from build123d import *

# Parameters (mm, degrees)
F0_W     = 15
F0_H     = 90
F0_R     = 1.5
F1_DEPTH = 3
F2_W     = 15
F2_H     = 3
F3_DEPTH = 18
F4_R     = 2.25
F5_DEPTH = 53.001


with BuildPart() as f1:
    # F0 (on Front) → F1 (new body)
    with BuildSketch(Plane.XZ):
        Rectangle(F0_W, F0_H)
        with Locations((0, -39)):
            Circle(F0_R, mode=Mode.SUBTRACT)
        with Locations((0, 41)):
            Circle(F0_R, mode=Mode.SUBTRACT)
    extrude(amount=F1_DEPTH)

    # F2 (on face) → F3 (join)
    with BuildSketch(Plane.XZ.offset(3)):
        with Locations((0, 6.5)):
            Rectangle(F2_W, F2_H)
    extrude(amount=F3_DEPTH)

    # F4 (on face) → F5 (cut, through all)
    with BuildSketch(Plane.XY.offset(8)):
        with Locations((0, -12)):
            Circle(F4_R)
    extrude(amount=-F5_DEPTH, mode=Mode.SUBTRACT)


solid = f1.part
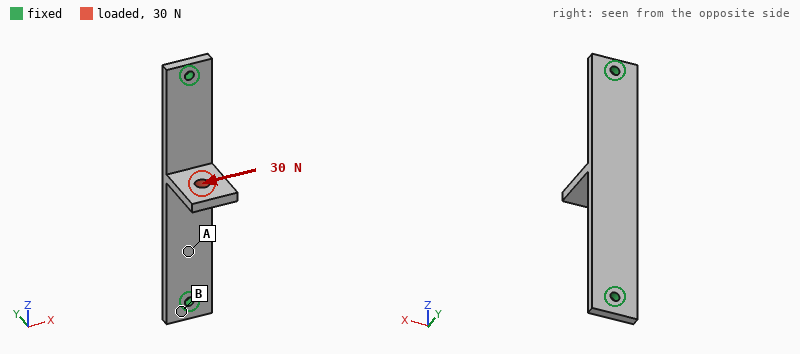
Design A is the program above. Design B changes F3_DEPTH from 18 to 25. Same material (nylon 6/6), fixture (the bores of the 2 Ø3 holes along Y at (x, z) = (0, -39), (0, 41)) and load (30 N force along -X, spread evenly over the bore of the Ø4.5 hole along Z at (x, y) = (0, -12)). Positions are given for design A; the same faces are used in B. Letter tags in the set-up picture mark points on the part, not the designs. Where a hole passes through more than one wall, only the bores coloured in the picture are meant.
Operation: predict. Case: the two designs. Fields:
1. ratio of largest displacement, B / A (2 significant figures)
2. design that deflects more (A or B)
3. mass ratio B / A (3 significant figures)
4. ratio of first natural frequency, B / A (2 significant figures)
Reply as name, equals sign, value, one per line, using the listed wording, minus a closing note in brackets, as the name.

ratio of largest displacement, B / A = 1.3
design that deflects more = B
mass ratio B / A = 1.07
ratio of first natural frequency, B / A = 0.93
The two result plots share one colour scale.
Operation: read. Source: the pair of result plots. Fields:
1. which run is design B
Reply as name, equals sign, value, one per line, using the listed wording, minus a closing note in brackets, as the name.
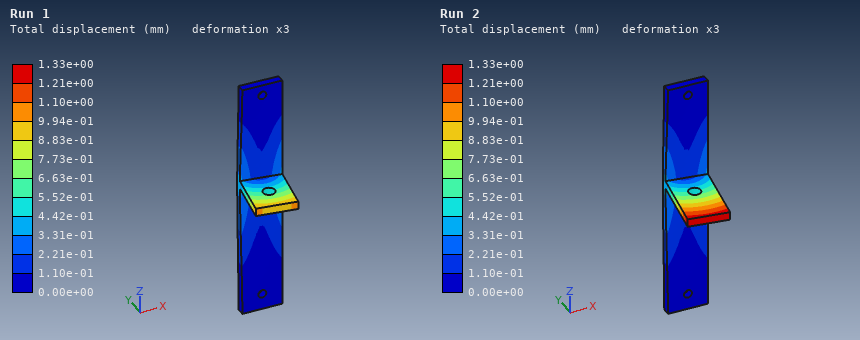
which run is design B = Run 2
